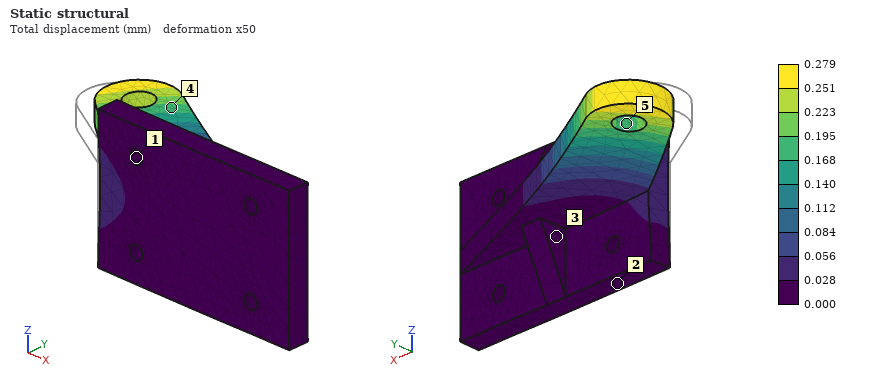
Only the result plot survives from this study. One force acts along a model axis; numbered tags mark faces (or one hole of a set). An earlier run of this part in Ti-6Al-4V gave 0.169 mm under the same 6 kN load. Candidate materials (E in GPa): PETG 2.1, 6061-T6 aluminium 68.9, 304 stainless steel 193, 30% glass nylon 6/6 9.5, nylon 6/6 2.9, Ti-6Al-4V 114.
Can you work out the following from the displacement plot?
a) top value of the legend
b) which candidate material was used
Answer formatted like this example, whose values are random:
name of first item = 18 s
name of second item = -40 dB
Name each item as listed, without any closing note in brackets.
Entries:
top value of the legend = 0.279 mm
which candidate material was used = 6061-T6 aluminium
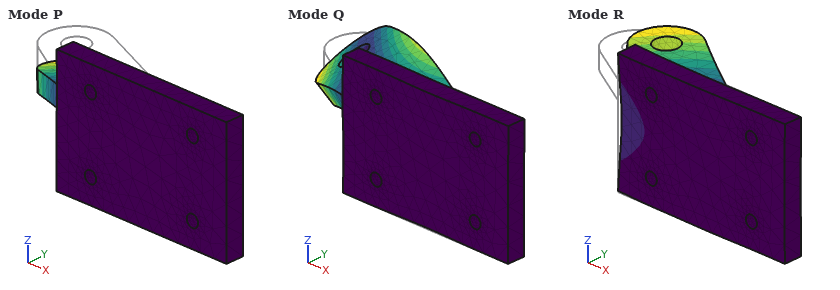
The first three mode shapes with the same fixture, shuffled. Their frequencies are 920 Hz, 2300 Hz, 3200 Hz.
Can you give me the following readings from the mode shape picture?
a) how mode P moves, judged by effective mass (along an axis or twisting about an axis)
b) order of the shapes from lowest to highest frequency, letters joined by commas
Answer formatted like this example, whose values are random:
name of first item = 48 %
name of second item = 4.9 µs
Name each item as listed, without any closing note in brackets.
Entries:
how mode P moves, judged by effective mass = along Z
order of the shapes from lowest to highest frequency, letters joined by commas = P, R, Q
